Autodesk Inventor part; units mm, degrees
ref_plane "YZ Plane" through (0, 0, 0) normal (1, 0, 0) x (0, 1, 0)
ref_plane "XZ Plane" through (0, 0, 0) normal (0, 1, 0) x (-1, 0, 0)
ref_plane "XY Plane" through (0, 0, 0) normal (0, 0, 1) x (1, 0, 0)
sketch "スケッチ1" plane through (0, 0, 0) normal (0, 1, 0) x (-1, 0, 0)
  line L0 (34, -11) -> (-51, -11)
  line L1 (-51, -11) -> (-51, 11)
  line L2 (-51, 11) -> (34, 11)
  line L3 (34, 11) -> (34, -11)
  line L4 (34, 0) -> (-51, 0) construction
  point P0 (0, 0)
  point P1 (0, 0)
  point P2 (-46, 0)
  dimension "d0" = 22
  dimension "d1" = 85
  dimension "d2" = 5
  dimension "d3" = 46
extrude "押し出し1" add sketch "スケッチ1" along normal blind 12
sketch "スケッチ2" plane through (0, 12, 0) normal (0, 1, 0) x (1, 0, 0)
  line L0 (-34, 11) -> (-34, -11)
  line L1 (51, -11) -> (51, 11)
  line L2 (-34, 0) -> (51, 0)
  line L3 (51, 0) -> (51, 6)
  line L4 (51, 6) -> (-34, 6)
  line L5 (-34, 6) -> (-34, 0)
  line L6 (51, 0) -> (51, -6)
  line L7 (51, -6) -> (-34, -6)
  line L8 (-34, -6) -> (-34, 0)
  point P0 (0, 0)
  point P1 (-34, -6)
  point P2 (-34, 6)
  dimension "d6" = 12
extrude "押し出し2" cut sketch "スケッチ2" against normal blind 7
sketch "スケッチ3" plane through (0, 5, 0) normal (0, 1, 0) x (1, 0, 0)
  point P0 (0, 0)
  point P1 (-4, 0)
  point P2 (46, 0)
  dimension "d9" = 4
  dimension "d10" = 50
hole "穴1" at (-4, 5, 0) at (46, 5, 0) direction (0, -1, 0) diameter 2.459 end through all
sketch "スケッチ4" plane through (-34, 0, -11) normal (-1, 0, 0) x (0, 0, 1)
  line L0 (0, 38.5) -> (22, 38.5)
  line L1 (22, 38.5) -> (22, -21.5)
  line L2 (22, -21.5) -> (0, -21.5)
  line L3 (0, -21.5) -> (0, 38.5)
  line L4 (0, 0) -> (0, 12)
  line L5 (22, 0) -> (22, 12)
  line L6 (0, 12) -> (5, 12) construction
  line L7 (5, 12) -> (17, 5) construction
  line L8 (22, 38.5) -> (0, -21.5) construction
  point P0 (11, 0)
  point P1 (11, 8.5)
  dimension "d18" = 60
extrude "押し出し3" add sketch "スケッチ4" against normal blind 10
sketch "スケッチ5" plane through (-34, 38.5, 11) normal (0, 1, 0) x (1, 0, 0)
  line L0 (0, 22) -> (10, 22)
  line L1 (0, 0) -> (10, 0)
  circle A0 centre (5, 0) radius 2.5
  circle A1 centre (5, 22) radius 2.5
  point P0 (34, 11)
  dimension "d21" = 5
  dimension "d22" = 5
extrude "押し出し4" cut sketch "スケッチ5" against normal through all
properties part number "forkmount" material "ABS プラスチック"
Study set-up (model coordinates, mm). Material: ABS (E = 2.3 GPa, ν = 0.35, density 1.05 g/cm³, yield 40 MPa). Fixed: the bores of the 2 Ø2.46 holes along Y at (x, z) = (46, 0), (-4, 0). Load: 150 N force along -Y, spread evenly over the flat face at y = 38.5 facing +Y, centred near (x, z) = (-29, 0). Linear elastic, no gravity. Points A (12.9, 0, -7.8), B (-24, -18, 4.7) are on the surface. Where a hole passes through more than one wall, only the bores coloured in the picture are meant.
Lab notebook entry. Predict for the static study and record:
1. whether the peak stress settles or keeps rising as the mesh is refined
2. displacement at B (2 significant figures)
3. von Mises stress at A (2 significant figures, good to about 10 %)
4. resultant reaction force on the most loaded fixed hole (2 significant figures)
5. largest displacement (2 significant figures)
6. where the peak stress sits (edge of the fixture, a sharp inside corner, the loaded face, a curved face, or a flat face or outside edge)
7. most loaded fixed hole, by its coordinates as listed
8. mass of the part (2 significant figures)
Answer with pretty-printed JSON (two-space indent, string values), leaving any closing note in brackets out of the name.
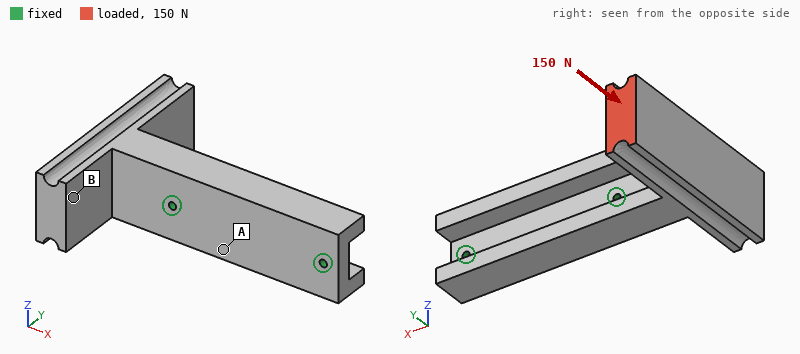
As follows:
{
  "whether the peak stress settles or keeps rising as the mesh is refined": "keeps rising",
  "displacement at B": "0.54 mm",
  "von Mises stress at A": "2.7 MPa",
  "resultant reaction force on the most loaded fixed hole": "240 N",
  "largest displacement": "0.86 mm",
  "where the peak stress sits": "edge of the fixture",
  "most loaded fixed hole, by its coordinates as listed": "(-4, 0)",
  "mass of the part": "27 g"
}
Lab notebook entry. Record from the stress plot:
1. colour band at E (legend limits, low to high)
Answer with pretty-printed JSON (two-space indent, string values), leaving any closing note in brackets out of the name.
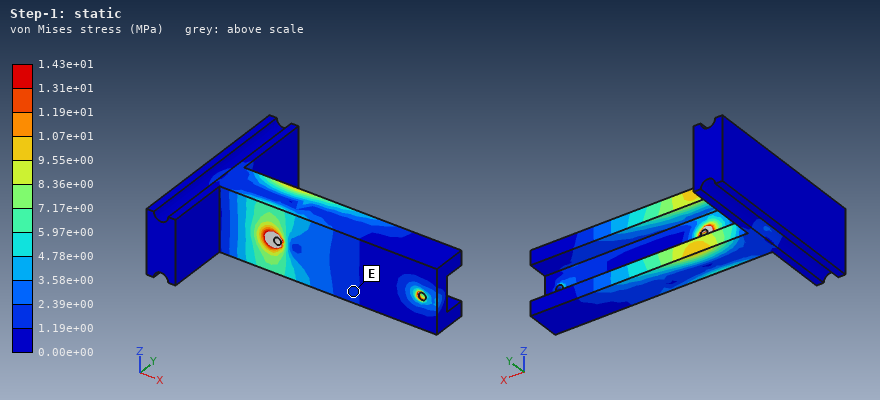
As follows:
{
  "colour band at E": "1.19e+00 to 2.39e+00 MPa"
}
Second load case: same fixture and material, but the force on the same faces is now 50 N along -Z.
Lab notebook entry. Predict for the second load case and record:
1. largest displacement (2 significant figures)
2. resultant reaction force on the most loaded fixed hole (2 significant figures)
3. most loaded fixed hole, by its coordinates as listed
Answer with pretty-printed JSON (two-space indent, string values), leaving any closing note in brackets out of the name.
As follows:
{
  "largest displacement": "1.1 mm",
  "resultant reaction force on the most loaded fixed hole": "72 N",
  "most loaded fixed hole, by its coordinates as listed": "(-4, 0)"
}
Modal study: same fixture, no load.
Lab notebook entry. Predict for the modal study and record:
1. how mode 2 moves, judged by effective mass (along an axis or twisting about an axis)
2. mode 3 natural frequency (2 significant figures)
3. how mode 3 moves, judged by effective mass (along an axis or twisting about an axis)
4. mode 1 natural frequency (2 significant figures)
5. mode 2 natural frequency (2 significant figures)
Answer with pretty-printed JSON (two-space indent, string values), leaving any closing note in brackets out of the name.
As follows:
{
  "how mode 2 moves, judged by effective mass": "along Y",
  "mode 3 natural frequency": "1300 Hz",
  "how mode 3 moves, judged by effective mass": "along Z",
  "mode 1 natural frequency": "570 Hz",
  "mode 2 natural frequency": "610 Hz"
}
